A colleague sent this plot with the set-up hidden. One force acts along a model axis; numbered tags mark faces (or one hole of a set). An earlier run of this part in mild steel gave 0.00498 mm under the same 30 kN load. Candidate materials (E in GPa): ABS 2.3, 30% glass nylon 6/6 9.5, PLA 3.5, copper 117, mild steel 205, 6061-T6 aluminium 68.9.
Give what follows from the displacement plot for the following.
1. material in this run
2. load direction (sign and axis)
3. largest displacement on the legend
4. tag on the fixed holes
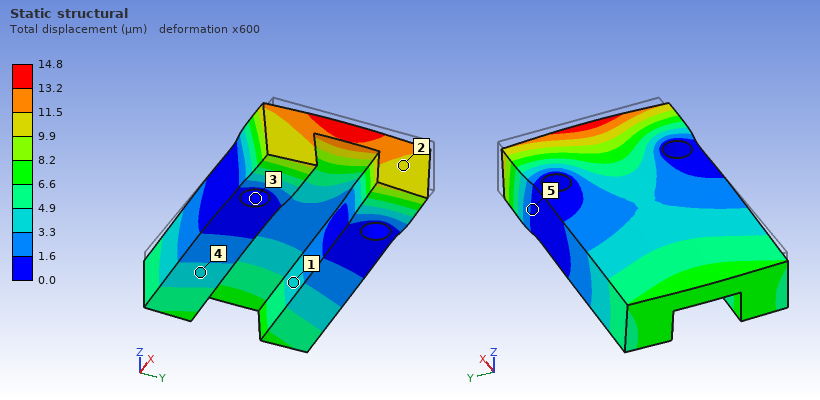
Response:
6061-T6 aluminium
-X
14.8 µm
3
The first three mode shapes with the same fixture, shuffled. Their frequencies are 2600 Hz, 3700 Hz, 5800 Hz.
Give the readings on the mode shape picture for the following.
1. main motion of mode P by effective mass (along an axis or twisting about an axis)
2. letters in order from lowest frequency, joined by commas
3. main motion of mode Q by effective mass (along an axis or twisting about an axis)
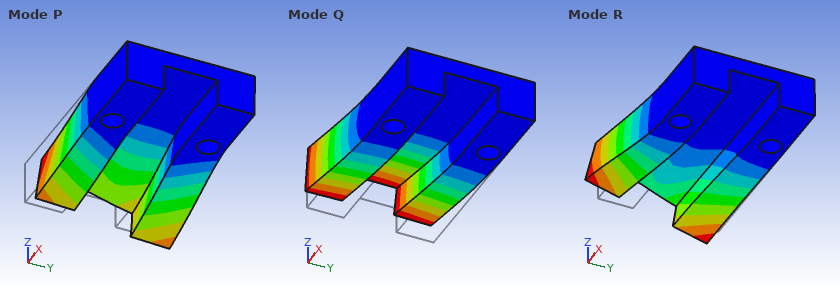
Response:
along Y
Q, R, P
along Z
